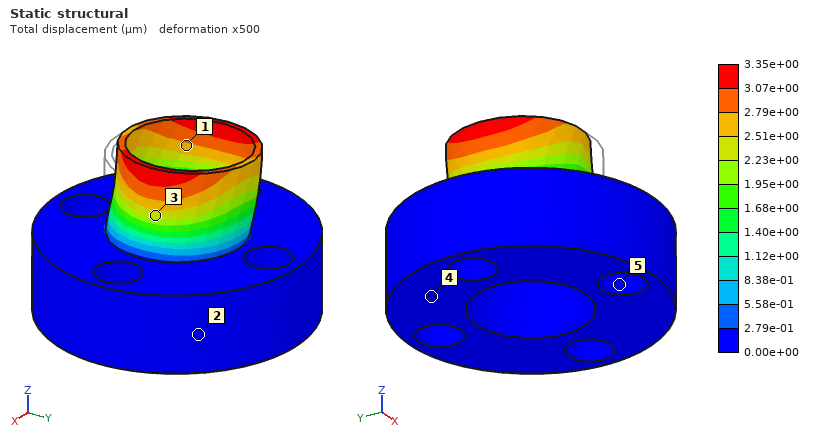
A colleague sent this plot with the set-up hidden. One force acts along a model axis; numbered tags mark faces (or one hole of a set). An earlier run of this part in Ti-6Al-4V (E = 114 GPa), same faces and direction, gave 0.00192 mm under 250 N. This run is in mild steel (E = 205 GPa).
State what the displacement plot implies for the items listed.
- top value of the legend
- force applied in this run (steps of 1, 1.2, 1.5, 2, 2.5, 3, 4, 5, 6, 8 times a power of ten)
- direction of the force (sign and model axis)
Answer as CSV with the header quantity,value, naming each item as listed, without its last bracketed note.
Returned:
quantity,value
top value of the legend,3.35e+00 µm
force applied in this run,800 N
direction of the force,-X
